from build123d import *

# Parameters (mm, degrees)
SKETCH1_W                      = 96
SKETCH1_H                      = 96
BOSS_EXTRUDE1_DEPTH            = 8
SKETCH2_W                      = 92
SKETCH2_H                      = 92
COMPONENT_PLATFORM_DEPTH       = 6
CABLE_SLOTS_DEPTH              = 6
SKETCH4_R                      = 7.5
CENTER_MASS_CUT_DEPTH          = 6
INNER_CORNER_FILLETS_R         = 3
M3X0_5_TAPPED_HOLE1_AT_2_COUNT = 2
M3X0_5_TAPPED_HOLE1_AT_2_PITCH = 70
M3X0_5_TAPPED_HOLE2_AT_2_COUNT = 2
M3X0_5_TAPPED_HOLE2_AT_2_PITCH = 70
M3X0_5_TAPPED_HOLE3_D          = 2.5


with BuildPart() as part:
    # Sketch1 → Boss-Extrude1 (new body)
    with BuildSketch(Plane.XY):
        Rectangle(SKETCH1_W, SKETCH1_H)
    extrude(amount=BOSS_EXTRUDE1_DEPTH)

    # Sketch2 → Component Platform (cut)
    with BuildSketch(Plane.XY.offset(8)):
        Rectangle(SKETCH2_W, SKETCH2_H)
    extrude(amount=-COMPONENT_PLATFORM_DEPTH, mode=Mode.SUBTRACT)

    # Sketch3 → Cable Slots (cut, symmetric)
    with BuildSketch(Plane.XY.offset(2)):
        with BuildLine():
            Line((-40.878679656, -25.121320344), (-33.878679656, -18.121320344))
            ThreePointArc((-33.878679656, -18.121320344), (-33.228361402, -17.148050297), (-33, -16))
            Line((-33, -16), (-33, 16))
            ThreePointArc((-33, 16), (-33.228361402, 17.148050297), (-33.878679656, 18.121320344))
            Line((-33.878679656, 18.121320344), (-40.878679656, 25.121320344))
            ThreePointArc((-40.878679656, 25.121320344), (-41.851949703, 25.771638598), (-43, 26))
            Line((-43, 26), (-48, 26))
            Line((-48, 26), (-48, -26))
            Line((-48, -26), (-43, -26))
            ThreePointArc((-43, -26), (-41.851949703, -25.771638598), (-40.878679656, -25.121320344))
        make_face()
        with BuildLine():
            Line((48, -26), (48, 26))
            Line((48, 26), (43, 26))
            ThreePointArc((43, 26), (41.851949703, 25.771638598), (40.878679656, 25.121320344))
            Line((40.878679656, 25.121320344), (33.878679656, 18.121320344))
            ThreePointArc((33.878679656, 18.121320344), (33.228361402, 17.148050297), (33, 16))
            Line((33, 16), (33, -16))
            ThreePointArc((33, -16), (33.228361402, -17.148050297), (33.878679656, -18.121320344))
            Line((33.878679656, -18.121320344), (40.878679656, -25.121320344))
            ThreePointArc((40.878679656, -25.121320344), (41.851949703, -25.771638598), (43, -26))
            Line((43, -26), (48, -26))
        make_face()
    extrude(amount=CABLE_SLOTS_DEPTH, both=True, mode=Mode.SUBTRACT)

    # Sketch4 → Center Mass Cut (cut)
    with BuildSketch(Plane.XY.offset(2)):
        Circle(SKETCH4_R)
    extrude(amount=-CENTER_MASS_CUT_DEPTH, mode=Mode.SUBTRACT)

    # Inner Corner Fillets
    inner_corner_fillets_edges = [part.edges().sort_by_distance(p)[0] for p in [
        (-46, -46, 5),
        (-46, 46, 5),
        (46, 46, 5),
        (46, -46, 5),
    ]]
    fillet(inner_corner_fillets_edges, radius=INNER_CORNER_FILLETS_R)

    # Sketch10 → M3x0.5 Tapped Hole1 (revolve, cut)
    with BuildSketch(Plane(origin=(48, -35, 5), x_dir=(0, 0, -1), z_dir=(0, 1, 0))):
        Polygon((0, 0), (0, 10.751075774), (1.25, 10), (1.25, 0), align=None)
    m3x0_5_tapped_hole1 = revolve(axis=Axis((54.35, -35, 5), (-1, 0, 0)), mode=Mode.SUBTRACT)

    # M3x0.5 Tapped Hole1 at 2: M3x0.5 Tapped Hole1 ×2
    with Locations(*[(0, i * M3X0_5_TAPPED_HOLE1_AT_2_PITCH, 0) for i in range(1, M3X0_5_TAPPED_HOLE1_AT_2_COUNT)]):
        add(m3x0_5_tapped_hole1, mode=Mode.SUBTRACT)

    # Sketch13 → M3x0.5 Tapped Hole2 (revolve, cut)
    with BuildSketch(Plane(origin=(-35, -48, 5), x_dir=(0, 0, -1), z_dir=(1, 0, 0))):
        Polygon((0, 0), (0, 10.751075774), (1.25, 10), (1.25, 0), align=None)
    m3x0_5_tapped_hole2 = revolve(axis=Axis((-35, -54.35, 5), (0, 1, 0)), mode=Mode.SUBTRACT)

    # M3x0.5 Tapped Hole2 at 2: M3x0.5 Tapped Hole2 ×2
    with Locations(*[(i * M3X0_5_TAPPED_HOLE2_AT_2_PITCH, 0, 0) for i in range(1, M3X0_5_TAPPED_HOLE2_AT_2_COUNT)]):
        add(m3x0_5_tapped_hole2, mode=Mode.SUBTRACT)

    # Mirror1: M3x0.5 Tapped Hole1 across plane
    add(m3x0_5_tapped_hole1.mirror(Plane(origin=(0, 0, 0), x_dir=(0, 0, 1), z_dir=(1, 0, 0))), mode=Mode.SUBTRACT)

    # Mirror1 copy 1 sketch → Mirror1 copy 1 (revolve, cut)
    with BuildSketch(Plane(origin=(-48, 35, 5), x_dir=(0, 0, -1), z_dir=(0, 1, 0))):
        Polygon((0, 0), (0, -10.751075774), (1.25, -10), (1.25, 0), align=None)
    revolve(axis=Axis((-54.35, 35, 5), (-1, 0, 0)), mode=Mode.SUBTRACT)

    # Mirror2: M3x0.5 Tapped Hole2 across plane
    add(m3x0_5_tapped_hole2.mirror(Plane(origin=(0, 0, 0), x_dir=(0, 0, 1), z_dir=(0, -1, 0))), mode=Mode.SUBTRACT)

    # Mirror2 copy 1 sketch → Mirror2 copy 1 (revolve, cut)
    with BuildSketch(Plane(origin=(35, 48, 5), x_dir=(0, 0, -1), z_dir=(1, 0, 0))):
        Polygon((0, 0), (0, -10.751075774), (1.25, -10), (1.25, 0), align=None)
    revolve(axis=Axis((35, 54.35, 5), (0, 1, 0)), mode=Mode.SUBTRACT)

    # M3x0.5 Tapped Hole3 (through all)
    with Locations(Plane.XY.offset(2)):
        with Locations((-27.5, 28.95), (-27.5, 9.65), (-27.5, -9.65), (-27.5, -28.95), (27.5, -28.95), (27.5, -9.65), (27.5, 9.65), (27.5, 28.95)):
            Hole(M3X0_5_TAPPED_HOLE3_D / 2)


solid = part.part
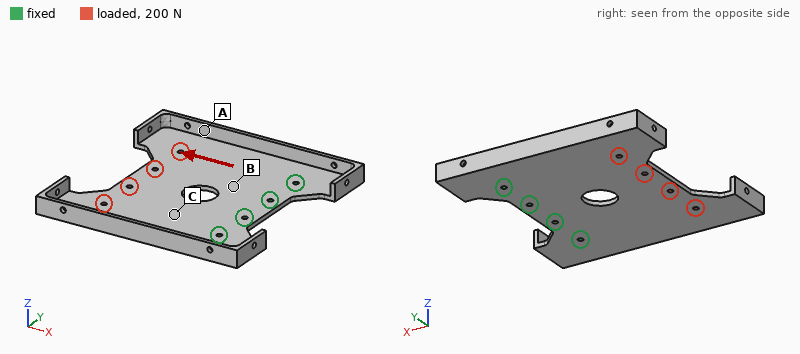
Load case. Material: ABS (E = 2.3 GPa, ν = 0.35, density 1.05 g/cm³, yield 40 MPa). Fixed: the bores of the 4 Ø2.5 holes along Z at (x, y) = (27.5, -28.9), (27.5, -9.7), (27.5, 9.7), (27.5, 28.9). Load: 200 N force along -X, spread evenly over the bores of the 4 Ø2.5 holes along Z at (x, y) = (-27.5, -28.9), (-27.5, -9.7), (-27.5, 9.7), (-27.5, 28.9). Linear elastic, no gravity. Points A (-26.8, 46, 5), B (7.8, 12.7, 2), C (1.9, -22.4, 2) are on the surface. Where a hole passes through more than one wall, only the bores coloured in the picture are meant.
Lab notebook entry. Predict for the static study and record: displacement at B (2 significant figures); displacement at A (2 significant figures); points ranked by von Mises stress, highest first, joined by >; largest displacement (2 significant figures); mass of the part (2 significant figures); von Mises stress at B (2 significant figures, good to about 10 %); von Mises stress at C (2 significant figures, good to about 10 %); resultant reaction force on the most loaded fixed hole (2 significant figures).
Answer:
15 µm
21 µm
B > C > A
49 µm
19 g
1.9 MPa
1.4 MPa
64 N
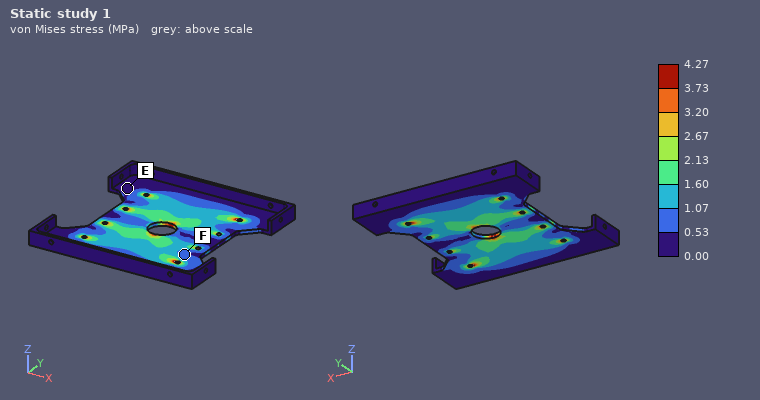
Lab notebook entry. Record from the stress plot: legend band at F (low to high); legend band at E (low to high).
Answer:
0.53 to 1.07 MPa
0.00 to 0.53 MPa
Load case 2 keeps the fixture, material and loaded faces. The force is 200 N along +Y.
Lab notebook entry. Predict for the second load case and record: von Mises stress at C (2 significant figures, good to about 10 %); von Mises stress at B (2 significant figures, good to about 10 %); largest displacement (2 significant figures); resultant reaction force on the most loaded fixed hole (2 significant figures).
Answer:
3.4 MPa
3.4 MPa
0.30 mm
190 N
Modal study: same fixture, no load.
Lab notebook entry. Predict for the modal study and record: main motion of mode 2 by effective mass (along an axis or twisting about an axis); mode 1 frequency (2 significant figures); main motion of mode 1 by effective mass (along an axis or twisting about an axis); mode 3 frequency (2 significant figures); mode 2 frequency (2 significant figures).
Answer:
twisting about X
110 Hz
along Z
370 Hz
140 Hz
